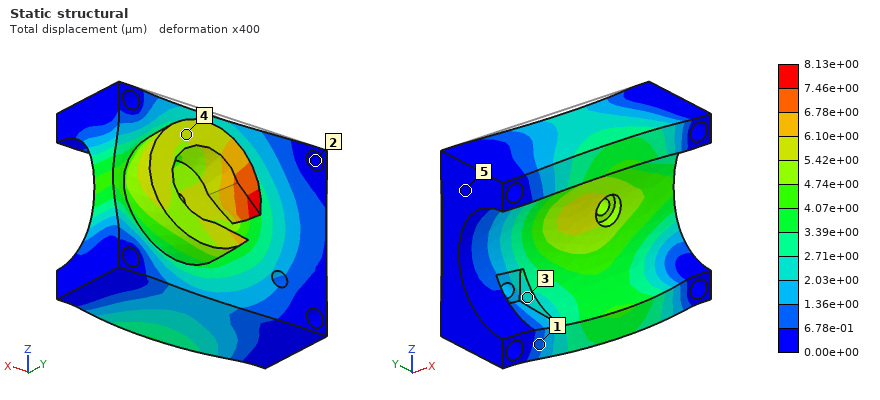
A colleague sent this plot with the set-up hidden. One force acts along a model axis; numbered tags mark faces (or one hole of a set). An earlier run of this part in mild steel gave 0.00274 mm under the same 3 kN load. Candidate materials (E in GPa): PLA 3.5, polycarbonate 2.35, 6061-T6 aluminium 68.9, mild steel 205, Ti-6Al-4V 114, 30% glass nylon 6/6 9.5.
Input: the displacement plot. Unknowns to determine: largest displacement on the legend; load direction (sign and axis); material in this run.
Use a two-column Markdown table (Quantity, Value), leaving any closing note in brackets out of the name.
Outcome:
| Quantity | Value |
|---|---|
| largest displacement on the legend | 8.13e+00 µm |
| load direction | -Y |
| material in this run | 6061-T6 aluminium |
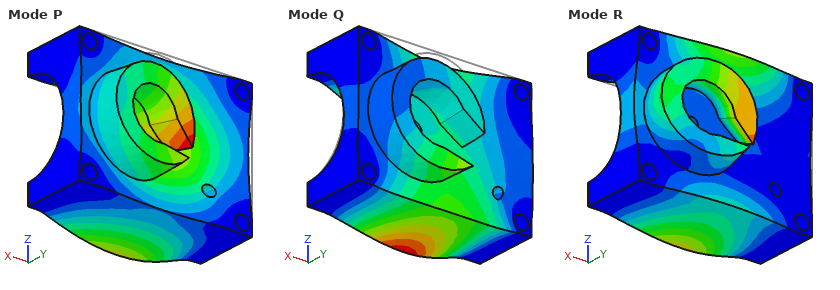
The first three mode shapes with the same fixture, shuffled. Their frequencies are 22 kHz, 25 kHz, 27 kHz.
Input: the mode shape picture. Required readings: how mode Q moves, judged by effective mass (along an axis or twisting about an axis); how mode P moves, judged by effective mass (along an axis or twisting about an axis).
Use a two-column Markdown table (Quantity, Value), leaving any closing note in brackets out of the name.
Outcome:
| Quantity | Value |
|---|---|
| how mode Q moves, judged by effective mass | along Z |
| how mode P moves, judged by effective mass | along Y |
